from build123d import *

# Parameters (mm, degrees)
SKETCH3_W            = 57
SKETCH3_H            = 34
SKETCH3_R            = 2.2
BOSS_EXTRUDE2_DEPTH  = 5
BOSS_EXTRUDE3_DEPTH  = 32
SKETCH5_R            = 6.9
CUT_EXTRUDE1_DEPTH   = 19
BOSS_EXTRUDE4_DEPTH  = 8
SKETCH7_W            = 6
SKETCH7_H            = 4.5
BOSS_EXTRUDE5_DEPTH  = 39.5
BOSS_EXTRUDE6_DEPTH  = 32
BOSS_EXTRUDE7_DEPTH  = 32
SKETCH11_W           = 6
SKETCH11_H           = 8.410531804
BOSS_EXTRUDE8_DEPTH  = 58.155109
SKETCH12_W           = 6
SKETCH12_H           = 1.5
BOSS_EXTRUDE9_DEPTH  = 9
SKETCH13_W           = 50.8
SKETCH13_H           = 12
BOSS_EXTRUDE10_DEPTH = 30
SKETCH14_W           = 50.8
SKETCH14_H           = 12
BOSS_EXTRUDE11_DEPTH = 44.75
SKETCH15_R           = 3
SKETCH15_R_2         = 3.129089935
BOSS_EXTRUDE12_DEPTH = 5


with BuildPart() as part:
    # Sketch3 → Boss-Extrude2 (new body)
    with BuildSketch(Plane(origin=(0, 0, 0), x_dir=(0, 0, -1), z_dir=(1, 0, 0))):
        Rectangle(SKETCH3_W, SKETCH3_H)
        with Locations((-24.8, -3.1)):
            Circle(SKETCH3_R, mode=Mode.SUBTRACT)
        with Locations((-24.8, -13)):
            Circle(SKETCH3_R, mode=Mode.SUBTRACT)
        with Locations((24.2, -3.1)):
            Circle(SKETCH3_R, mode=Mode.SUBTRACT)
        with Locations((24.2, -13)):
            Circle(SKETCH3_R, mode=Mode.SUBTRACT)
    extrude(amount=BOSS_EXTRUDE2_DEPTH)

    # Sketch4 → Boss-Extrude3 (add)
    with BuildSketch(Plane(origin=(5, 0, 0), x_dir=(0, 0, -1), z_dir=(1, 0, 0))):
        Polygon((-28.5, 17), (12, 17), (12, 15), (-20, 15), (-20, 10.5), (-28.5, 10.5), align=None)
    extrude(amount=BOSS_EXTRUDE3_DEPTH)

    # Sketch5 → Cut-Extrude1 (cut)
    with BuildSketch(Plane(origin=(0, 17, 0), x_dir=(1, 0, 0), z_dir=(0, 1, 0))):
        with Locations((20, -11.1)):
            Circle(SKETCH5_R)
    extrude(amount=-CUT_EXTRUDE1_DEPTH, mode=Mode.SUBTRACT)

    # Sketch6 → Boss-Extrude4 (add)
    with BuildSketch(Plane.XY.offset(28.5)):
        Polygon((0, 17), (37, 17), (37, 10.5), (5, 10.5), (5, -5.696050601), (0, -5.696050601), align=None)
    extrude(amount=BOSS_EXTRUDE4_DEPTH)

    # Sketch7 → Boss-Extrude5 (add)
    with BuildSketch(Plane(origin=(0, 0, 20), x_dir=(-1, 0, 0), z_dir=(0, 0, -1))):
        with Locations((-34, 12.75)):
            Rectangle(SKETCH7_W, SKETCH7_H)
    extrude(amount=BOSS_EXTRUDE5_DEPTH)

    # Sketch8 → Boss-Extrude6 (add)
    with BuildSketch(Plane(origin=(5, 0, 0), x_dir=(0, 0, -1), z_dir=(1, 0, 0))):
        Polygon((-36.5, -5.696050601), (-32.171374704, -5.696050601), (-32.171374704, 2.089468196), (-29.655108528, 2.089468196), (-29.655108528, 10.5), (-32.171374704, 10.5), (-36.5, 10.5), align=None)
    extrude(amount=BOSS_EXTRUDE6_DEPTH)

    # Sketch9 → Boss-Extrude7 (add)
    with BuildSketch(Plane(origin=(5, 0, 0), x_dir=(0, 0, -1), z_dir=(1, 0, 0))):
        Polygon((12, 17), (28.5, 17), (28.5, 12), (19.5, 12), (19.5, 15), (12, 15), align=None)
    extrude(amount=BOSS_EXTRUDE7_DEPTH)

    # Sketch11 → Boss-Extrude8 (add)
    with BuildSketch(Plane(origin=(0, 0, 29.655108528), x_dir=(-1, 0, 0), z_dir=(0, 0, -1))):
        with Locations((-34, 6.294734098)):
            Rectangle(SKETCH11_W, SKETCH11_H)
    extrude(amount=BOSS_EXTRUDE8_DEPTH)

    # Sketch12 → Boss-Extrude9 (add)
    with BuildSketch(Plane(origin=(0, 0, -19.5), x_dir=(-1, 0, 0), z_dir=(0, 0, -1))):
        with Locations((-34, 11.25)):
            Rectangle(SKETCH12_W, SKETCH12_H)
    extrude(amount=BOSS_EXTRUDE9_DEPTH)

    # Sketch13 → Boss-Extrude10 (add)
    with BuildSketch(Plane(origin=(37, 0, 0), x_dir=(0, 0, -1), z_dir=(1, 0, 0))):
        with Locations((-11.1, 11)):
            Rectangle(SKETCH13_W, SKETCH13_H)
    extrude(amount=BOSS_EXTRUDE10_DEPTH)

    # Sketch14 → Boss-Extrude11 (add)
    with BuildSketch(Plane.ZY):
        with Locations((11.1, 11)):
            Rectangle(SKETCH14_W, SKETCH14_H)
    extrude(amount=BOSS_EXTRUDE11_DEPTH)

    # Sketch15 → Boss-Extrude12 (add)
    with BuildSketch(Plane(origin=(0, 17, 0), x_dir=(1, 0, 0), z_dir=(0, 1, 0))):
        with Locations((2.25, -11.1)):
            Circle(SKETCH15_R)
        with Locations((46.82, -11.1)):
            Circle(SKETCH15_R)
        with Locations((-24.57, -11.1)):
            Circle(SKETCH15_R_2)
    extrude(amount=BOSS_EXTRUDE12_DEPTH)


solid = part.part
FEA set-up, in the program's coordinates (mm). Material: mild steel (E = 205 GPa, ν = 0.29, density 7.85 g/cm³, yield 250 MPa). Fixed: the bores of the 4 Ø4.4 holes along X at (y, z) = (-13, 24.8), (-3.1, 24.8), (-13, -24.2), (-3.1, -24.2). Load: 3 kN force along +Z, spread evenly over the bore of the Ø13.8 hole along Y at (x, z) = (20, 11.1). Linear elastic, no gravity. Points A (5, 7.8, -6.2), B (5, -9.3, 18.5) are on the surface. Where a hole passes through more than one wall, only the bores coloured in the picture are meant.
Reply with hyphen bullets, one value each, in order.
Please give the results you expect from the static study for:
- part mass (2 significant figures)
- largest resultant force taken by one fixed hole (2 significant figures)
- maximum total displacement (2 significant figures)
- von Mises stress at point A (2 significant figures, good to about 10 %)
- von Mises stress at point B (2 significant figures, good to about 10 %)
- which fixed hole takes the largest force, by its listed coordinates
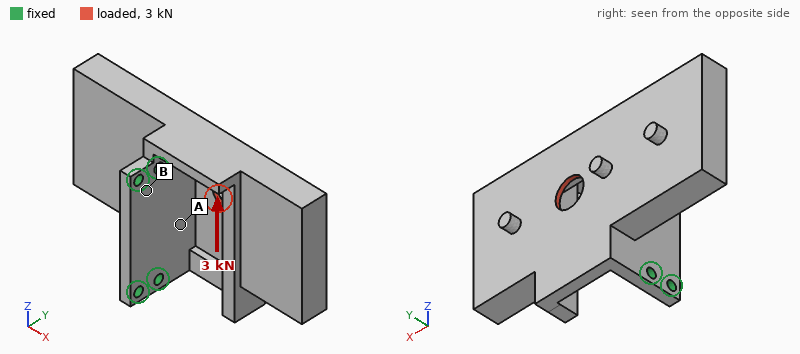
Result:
- 550 g
- 2.1 kN
- 59 µm
- 44 MPa
- 13 MPa
- (-3.1, 24.8)
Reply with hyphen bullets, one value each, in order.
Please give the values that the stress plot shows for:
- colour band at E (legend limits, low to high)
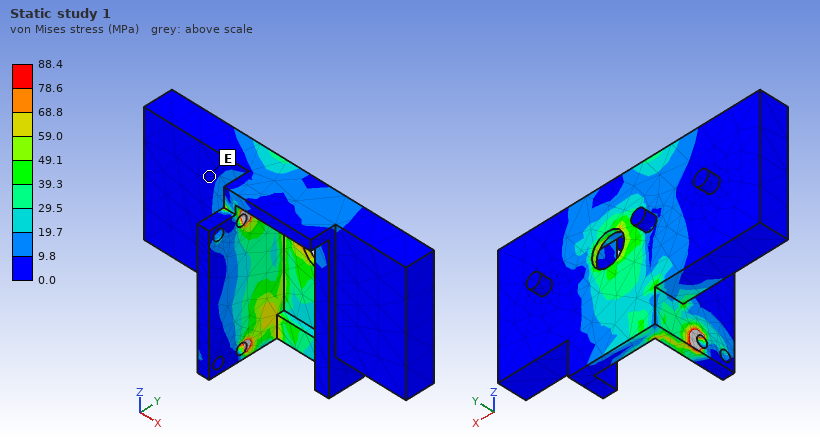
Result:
- 0.0 to 9.8 MPa
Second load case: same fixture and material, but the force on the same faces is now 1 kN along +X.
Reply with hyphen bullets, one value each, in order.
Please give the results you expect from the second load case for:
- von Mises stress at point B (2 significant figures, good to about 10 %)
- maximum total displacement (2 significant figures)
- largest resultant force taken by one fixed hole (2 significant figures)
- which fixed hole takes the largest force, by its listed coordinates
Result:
- 20 MPa
- 87 µm
- 1.0 kN
- (-3.1, 24.8)
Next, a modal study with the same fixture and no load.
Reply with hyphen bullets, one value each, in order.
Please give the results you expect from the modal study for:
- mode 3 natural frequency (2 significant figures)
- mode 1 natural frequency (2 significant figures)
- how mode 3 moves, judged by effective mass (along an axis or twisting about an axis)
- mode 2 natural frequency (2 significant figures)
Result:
- 2100 Hz
- 640 Hz
- along Y
- 1700 Hz
